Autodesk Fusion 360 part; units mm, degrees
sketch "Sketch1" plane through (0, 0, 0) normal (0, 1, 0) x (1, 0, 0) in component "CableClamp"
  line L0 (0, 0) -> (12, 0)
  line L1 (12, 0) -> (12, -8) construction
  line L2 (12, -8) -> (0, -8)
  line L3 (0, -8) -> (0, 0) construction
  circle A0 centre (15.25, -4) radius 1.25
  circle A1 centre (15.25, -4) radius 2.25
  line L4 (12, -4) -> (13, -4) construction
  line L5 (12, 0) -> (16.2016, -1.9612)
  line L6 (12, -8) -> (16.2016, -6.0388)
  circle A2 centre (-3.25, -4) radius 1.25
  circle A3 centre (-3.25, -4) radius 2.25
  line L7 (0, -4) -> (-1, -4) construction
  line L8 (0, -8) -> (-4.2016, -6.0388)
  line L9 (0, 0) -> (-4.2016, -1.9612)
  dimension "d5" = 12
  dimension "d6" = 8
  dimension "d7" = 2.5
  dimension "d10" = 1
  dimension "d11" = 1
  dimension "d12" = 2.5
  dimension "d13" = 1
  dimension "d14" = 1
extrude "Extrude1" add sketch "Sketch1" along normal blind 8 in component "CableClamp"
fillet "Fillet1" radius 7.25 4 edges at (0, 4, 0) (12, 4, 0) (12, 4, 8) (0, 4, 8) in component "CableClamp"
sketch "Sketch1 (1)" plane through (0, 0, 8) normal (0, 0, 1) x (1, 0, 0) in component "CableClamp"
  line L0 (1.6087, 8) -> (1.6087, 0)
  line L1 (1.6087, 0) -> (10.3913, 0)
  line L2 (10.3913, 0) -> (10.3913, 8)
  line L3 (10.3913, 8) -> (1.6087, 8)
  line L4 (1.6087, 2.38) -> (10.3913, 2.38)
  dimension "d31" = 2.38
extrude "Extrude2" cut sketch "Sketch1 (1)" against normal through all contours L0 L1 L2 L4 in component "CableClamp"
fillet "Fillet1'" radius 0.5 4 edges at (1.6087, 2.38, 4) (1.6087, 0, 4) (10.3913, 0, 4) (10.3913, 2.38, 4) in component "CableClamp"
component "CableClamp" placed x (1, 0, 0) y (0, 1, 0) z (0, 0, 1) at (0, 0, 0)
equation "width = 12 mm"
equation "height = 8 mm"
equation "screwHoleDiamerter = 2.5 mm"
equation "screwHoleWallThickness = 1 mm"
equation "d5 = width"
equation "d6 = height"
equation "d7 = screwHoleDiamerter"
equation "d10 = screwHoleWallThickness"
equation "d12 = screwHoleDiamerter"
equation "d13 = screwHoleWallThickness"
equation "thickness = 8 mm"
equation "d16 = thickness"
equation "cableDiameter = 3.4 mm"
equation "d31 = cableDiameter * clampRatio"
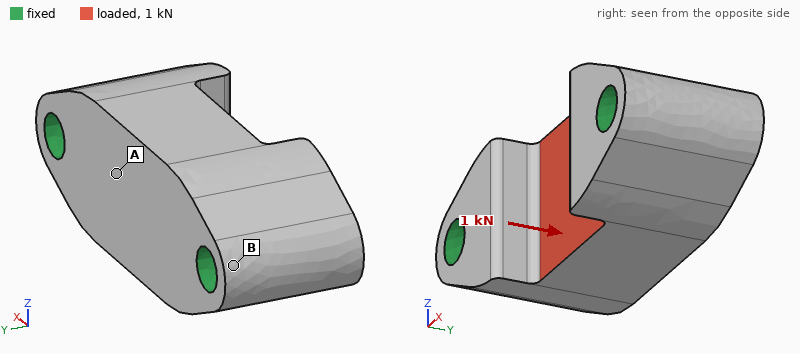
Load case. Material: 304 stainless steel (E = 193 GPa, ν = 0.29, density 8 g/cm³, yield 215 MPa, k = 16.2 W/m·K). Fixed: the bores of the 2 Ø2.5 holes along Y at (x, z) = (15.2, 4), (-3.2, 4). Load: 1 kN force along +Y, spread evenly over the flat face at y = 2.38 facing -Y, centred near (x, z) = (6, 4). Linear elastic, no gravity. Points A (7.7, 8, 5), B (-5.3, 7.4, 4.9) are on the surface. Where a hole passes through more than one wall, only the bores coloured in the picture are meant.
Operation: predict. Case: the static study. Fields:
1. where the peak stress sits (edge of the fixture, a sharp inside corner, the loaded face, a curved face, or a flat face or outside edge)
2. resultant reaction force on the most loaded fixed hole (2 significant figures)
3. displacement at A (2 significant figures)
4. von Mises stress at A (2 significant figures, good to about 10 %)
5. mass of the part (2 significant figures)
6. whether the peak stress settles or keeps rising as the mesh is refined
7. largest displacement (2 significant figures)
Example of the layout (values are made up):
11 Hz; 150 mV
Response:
edge of the fixture; 510 N; 1.4 µm; 24 MPa; 7.9 g; keeps rising; 1.9 µm
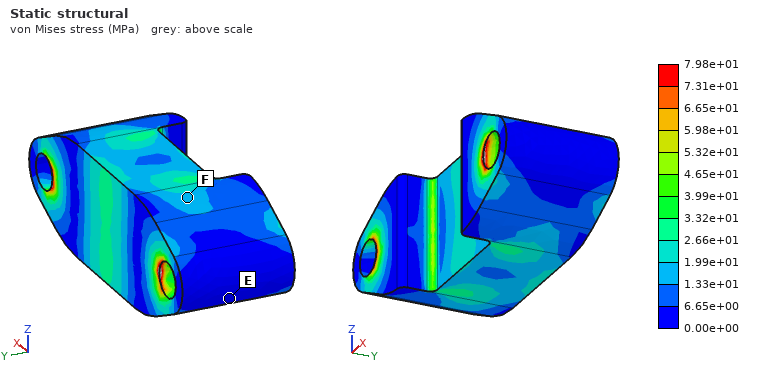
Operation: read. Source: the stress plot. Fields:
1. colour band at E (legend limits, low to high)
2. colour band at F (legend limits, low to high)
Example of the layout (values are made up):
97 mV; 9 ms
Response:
0.00e+00 to 6.65e+00 MPa; 1.33e+01 to 1.99e+01 MPa
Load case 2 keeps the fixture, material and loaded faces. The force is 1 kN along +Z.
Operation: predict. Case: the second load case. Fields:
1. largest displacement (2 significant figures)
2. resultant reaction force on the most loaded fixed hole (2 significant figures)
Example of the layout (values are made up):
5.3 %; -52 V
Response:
3.6 µm; 500 N
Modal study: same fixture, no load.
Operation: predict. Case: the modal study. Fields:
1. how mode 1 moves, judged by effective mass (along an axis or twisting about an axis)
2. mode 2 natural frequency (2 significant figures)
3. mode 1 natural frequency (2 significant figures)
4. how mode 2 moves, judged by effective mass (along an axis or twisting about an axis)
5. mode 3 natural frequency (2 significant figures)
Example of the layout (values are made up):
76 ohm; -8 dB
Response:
along Z; 68 kHz; 58 kHz; along Y; 85 kHz
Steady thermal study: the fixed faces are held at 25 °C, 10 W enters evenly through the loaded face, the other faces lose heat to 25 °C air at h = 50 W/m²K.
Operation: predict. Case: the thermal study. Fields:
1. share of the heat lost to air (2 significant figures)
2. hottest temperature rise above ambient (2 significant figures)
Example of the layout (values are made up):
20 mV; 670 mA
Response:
5.1 %; 59 K
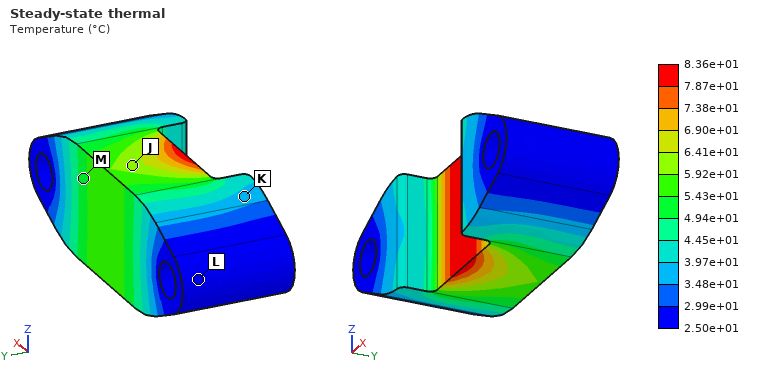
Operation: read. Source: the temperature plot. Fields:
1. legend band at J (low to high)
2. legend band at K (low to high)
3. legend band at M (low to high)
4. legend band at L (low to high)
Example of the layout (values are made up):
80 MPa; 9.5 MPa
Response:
5.92e+01 to 6.41e+01 °C; 3.48e+01 to 3.97e+01 °C; 4.94e+01 to 5.43e+01 °C; 2.50e+01 to 2.99e+01 °C
